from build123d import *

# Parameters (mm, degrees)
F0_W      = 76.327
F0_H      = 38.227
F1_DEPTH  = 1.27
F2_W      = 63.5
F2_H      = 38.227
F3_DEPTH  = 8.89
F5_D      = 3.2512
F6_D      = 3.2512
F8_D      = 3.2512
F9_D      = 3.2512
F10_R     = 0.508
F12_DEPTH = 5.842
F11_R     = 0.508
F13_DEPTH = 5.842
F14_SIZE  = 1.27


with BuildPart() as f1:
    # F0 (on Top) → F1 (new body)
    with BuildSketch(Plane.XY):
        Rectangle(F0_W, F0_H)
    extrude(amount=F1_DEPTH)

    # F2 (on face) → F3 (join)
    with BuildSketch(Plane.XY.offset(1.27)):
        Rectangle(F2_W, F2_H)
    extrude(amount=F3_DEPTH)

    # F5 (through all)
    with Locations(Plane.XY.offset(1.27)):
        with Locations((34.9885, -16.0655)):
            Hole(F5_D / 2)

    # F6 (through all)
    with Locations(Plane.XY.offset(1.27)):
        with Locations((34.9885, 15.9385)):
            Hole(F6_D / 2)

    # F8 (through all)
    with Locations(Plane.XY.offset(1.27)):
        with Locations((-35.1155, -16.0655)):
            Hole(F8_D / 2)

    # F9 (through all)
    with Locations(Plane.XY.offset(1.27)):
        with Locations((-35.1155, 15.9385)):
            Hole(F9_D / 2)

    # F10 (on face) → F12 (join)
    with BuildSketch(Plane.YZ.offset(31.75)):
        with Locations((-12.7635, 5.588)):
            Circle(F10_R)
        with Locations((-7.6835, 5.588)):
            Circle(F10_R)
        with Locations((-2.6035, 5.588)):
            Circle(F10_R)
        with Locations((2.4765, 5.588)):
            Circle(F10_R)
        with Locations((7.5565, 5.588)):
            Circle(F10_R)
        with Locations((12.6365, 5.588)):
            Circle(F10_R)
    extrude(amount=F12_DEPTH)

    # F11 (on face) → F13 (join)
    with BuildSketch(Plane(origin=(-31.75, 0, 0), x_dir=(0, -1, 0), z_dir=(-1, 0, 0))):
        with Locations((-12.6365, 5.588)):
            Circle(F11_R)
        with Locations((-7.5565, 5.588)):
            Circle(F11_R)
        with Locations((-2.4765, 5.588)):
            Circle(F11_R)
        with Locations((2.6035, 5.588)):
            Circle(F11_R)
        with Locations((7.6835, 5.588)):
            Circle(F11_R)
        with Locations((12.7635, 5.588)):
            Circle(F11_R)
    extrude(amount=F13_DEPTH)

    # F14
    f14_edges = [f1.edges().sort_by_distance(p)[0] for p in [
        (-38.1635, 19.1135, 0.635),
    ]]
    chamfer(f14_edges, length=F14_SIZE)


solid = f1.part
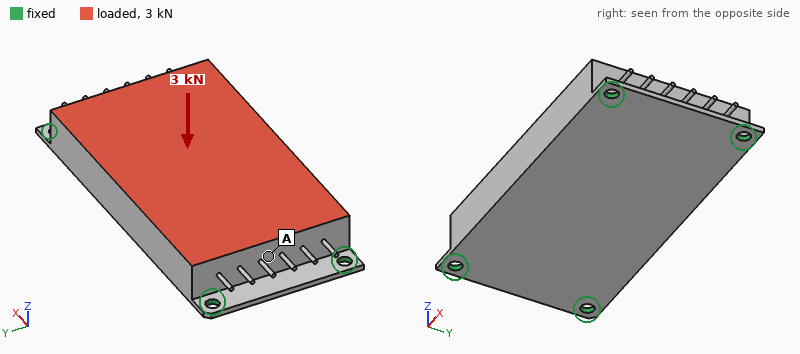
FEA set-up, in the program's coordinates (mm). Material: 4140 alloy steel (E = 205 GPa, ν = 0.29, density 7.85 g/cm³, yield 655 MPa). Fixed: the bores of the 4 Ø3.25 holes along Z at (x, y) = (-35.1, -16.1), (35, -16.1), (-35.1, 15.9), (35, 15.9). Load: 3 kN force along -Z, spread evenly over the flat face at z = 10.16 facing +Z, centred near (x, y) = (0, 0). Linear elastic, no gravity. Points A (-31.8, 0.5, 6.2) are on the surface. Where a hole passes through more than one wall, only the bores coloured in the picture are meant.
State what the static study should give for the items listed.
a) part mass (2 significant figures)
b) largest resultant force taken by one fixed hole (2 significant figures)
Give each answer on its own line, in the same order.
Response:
200 g
1.2 kN
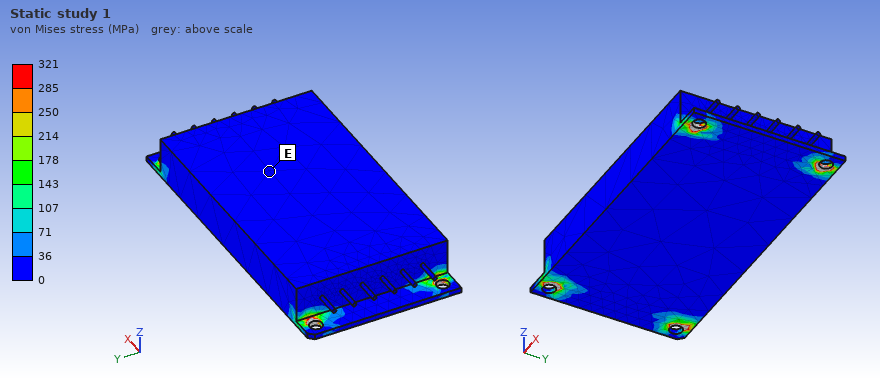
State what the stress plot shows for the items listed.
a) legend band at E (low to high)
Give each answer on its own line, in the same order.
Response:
0 to 36 MPa
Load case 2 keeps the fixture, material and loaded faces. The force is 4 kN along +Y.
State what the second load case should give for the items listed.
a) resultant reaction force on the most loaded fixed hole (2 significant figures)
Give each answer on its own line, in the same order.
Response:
1.4 kN
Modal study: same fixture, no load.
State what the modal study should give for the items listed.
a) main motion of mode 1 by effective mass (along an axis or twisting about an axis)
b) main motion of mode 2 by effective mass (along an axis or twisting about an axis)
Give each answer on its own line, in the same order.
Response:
along Z
along Y
